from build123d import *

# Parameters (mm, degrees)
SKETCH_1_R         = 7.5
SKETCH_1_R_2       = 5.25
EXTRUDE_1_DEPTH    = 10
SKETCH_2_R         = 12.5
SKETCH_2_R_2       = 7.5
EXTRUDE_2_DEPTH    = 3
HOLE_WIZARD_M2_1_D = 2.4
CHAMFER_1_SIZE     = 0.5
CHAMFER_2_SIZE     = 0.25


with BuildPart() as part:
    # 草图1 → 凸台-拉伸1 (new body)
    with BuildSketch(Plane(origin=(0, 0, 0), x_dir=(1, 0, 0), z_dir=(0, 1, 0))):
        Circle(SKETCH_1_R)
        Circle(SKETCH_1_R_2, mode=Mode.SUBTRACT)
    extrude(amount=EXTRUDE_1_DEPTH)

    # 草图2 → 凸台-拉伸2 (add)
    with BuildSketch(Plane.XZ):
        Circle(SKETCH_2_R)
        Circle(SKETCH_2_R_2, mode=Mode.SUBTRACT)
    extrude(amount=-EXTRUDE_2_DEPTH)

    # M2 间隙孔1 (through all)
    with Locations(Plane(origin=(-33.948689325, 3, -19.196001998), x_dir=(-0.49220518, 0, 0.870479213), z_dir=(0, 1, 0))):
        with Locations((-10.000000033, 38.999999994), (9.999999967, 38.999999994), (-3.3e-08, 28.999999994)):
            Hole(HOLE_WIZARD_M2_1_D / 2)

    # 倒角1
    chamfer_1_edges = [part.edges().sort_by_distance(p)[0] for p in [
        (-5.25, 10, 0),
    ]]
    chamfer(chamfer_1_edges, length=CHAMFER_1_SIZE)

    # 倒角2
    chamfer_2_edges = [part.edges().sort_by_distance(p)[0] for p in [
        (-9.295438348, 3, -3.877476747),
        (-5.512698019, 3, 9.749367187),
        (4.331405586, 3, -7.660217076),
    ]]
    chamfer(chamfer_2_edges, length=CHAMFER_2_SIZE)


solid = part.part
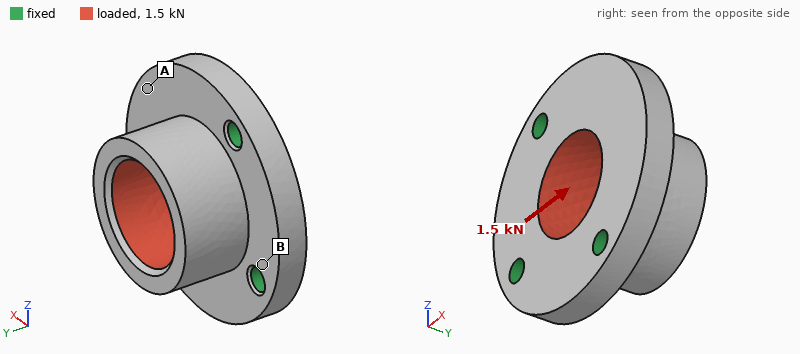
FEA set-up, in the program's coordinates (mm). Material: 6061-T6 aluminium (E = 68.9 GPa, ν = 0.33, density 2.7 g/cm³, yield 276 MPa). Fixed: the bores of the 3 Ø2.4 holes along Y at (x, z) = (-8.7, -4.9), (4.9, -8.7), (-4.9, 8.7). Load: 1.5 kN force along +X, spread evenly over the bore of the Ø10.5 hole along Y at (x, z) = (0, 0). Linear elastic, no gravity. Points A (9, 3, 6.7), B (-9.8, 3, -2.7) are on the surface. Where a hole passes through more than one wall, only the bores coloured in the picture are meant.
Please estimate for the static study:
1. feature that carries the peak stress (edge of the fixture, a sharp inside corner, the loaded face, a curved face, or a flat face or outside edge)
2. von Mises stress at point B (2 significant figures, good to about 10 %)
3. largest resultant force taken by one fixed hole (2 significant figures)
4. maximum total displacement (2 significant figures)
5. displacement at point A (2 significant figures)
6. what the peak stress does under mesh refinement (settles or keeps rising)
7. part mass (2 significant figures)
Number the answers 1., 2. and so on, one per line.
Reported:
1. edge of the fixture
2. 23 MPa
3. 600 N
4. 24 µm
5. 21 µm
6. keeps rising
7. 4.9 g
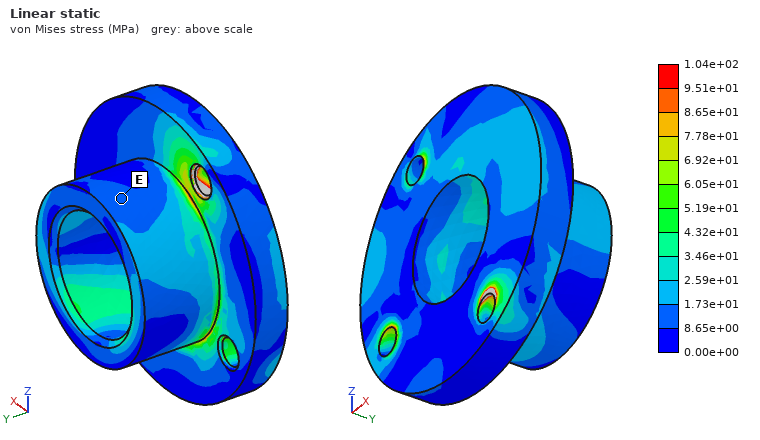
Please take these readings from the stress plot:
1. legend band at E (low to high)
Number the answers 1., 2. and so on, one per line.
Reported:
1. 8.65e+00 to 1.73e+01 MPa
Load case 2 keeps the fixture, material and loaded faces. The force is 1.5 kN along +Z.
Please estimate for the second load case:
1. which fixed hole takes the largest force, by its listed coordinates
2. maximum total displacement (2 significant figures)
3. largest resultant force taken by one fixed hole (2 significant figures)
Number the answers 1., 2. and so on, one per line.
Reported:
1. (4.9, -8.7)
2. 15 µm
3. 660 N
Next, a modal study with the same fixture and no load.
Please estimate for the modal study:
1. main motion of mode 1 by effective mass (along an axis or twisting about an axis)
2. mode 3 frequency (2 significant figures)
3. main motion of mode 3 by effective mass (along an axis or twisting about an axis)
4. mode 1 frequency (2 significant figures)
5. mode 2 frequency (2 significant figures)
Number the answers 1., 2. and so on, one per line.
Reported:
1. along Y
2. 44 kHz
3. along Z
4. 17 kHz
5. 39 kHz
